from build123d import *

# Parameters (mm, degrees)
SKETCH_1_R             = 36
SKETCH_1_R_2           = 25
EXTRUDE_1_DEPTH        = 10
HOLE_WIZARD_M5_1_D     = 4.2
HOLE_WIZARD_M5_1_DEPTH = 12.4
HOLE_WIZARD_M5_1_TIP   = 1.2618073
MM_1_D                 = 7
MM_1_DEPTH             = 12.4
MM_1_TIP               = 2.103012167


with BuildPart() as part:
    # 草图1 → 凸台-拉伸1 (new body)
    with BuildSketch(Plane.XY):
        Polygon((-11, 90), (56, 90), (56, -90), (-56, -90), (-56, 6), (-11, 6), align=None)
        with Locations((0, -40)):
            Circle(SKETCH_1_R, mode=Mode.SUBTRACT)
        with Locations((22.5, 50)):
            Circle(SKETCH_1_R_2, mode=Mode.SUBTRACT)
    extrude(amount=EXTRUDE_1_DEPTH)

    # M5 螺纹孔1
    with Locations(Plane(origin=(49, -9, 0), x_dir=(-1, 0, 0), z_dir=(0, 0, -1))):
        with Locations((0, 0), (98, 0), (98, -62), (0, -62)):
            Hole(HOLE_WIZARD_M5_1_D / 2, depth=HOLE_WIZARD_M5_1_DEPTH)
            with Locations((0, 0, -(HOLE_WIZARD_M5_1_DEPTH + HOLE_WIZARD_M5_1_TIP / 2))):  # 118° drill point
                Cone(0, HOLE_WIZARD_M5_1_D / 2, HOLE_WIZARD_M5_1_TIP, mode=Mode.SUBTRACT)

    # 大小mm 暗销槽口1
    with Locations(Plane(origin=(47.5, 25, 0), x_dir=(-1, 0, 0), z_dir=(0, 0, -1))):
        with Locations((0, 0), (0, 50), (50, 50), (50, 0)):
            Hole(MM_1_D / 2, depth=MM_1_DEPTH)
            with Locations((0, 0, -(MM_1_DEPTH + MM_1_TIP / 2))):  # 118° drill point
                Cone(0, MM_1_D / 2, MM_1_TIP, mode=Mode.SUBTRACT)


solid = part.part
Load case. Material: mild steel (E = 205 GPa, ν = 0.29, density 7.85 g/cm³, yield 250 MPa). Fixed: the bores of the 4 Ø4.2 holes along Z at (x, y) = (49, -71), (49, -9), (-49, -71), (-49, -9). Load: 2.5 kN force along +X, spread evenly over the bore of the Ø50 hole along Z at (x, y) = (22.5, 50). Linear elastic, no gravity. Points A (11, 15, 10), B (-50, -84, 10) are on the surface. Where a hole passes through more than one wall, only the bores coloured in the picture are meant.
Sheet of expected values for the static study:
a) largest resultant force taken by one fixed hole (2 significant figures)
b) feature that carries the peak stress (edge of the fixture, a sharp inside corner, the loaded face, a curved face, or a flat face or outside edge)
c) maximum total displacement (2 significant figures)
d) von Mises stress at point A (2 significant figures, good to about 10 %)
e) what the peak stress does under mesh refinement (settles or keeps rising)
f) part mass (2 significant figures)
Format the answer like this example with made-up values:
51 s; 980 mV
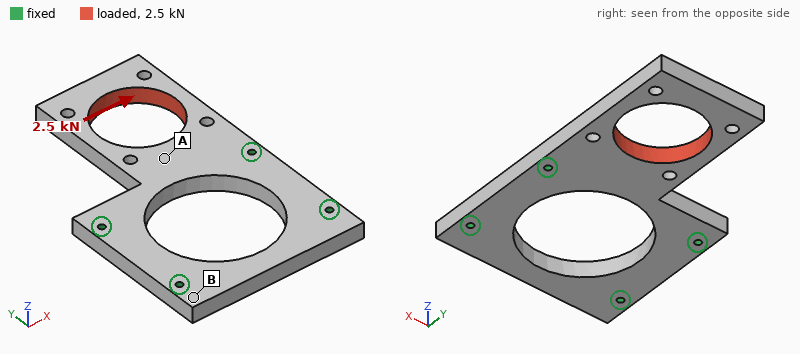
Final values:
2.0 kN; edge of the fixture; 50 µm; 14 MPa; keeps rising; 800 g
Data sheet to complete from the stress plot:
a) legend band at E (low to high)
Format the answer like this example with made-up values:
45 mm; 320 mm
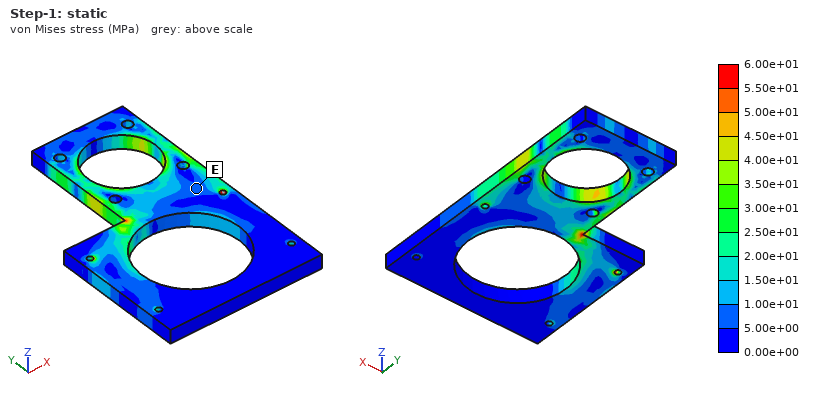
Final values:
5.00e+00 to 1.00e+01 MPa
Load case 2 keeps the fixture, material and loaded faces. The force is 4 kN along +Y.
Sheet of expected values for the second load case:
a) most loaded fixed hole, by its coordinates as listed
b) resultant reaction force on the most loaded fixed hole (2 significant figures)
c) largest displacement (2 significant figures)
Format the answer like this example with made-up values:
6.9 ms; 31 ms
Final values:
(49, -9); 2.5 kN; 16 µm
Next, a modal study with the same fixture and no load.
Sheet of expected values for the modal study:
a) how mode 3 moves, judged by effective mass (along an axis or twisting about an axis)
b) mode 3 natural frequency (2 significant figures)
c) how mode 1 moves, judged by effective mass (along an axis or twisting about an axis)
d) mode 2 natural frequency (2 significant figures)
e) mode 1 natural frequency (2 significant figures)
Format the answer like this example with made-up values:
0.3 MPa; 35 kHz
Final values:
along X; 2500 Hz; along Z; 2000 Hz; 670 Hz
